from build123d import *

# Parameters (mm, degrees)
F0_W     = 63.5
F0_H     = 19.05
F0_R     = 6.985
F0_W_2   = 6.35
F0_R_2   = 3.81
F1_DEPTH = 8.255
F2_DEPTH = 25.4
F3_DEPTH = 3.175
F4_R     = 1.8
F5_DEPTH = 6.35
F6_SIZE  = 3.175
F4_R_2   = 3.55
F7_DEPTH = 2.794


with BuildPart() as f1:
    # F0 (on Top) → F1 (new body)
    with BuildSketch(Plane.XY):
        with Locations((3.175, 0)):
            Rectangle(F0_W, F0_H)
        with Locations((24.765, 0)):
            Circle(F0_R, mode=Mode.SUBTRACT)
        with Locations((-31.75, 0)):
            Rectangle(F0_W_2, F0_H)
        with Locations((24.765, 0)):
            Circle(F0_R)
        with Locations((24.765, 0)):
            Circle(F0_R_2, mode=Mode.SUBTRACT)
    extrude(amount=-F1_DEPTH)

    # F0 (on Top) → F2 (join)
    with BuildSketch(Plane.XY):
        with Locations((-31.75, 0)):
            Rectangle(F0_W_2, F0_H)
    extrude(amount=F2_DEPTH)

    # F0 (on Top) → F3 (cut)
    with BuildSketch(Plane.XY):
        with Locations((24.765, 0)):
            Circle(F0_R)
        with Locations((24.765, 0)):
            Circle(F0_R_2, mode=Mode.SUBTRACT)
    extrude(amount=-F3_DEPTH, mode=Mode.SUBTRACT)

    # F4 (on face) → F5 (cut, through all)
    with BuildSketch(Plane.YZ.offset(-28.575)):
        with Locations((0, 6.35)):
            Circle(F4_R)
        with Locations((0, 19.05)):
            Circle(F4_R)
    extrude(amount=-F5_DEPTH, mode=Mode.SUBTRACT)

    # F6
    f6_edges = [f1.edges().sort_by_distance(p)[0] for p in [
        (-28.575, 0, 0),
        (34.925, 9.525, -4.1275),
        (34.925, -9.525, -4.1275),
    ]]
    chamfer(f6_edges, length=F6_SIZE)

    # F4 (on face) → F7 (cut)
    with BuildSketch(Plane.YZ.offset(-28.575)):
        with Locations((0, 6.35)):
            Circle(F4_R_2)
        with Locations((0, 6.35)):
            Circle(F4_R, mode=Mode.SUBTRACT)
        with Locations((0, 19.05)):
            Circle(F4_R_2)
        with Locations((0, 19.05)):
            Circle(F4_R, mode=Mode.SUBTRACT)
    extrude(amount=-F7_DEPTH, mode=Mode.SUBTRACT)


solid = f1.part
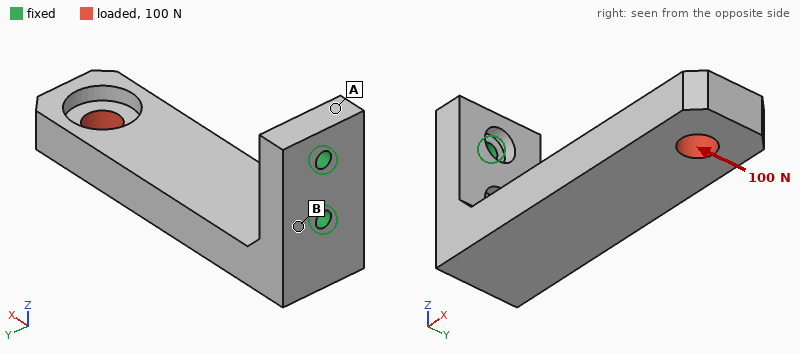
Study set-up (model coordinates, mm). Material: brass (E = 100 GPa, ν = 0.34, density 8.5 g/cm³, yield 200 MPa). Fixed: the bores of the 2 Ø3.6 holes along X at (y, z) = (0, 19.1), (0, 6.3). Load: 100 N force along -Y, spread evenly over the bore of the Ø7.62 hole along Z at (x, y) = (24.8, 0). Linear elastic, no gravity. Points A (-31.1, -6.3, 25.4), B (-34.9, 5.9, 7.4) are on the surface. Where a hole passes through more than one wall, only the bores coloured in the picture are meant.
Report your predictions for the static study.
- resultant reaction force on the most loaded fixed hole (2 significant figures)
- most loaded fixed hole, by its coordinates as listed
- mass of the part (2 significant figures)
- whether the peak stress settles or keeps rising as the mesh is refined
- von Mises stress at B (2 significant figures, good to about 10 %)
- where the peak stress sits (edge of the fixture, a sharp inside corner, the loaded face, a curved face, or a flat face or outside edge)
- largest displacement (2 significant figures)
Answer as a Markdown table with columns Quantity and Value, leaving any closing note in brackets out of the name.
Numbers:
| Quantity | Value |
|---|---|
| resultant reaction force on the most loaded fixed hole | 140 N |
| most loaded fixed hole, by its coordinates as listed | (0, 6.3) |
| mass of the part | 110 g |
| whether the peak stress settles or keeps rising as the mesh is refined | keeps rising |
| von Mises stress at B | 23 MPa |
| where the peak stress sits | edge of the fixture |
| largest displacement | 0.11 mm |
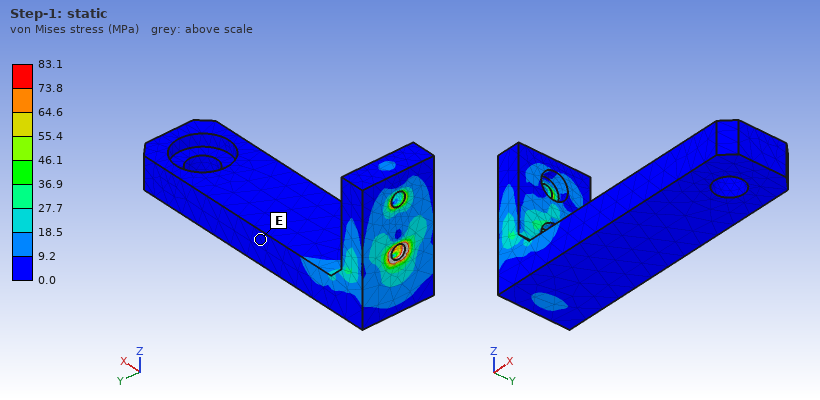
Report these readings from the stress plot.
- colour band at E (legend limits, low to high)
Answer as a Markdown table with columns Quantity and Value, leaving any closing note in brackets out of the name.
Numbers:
| Quantity | Value |
|---|---|
| colour band at E | 0.0 to 9.2 MPa |
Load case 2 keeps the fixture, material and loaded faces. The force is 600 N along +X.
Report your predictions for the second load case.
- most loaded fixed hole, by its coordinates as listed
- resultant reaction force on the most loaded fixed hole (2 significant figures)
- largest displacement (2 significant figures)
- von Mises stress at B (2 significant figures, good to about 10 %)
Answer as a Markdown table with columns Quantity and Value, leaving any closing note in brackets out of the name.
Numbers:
| Quantity | Value |
|---|---|
| most loaded fixed hole, by its coordinates as listed | (0, 6.3) |
| resultant reaction force on the most loaded fixed hole | 980 N |
| largest displacement | 0.13 mm |
| von Mises stress at B | 32 MPa |
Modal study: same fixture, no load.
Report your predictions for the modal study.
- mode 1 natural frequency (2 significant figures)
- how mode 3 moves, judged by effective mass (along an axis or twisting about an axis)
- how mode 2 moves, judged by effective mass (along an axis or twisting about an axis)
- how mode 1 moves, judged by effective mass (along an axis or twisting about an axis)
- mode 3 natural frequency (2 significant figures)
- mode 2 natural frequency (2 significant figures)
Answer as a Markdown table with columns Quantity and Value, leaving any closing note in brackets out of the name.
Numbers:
| Quantity | Value |
|---|---|
| mode 1 natural frequency | 730 Hz |
| how mode 3 moves, judged by effective mass | along X |
| how mode 2 moves, judged by effective mass | along Y |
| how mode 1 moves, judged by effective mass | along Z |
| mode 3 natural frequency | 4100 Hz |
| mode 2 natural frequency | 870 Hz |
